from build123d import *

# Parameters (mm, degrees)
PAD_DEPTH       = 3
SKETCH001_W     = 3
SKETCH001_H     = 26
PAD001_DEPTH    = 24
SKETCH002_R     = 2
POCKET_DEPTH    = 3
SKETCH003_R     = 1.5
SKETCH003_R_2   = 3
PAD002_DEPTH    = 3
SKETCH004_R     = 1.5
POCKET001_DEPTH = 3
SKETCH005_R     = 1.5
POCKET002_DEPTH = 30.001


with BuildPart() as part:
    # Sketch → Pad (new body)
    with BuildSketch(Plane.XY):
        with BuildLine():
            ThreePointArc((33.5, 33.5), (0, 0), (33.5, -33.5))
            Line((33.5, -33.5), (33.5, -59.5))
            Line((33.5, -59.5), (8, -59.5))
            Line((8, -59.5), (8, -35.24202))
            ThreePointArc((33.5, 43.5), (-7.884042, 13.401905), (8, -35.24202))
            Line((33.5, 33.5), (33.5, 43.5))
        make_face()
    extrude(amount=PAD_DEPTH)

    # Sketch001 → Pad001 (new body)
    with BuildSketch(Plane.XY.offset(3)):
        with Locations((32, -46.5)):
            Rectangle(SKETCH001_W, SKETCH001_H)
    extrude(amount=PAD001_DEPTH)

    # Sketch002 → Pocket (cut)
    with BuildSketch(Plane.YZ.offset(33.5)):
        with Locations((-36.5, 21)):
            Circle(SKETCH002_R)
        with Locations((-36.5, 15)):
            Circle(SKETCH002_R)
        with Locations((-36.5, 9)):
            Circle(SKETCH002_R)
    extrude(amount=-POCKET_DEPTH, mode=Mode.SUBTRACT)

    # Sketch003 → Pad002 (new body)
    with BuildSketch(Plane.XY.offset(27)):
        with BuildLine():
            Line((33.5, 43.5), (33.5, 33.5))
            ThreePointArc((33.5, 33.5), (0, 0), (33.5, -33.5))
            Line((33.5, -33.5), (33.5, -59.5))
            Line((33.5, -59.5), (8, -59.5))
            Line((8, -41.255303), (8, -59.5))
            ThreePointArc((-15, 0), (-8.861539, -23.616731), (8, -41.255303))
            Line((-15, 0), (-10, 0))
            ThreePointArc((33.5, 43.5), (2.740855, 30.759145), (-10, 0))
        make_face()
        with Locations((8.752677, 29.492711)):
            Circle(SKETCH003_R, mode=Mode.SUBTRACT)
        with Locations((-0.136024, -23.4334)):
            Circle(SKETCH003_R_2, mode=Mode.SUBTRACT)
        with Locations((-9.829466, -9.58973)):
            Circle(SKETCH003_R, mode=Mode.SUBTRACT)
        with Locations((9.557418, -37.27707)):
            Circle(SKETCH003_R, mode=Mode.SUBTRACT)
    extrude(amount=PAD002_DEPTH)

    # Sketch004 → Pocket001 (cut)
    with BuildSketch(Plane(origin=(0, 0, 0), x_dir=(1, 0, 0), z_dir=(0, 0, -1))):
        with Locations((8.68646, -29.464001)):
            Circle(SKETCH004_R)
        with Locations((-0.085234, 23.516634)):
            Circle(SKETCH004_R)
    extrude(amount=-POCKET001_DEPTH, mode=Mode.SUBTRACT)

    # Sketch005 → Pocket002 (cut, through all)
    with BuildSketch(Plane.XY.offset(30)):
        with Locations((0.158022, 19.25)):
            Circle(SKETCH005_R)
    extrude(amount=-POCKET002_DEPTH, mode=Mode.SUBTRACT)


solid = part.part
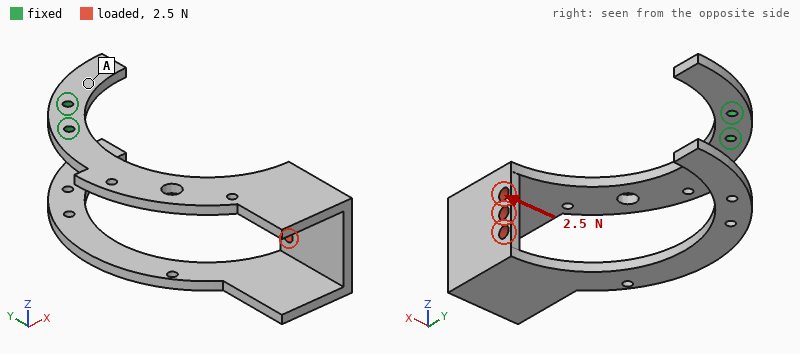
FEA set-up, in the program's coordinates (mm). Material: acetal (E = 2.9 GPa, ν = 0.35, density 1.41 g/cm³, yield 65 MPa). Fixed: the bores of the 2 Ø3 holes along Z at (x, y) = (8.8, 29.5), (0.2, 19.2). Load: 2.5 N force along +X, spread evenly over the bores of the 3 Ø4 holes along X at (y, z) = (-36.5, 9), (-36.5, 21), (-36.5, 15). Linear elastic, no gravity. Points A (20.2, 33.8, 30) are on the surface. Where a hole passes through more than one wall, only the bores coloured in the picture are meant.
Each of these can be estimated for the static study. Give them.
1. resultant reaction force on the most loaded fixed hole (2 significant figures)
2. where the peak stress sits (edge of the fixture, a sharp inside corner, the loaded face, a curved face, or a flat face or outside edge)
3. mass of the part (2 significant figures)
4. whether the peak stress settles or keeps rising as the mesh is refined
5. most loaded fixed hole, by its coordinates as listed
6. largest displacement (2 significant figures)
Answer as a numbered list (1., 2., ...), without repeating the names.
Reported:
1. 7.6 N
2. edge of the fixture
3. 17 g
4. keeps rising
5. (0.2, 19.2)
6. 1.4 mm
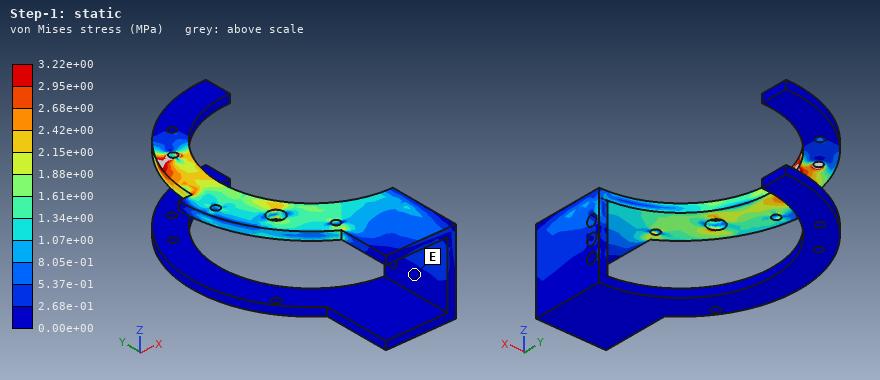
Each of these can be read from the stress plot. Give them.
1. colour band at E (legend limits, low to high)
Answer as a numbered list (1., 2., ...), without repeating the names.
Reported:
1. 0.00e+00 to 2.68e-01 MPa
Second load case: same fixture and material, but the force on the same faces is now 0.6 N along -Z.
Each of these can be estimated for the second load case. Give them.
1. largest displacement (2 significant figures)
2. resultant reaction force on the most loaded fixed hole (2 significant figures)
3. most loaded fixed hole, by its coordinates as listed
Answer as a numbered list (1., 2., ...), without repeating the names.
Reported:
1. 1.4 mm
2. 0.81 N
3. (0.2, 19.2)
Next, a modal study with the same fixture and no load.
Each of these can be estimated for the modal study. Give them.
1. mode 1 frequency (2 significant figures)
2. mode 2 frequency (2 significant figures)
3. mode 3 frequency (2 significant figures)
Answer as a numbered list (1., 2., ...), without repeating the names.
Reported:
1. 34 Hz
2. 51 Hz
3. 65 Hz
